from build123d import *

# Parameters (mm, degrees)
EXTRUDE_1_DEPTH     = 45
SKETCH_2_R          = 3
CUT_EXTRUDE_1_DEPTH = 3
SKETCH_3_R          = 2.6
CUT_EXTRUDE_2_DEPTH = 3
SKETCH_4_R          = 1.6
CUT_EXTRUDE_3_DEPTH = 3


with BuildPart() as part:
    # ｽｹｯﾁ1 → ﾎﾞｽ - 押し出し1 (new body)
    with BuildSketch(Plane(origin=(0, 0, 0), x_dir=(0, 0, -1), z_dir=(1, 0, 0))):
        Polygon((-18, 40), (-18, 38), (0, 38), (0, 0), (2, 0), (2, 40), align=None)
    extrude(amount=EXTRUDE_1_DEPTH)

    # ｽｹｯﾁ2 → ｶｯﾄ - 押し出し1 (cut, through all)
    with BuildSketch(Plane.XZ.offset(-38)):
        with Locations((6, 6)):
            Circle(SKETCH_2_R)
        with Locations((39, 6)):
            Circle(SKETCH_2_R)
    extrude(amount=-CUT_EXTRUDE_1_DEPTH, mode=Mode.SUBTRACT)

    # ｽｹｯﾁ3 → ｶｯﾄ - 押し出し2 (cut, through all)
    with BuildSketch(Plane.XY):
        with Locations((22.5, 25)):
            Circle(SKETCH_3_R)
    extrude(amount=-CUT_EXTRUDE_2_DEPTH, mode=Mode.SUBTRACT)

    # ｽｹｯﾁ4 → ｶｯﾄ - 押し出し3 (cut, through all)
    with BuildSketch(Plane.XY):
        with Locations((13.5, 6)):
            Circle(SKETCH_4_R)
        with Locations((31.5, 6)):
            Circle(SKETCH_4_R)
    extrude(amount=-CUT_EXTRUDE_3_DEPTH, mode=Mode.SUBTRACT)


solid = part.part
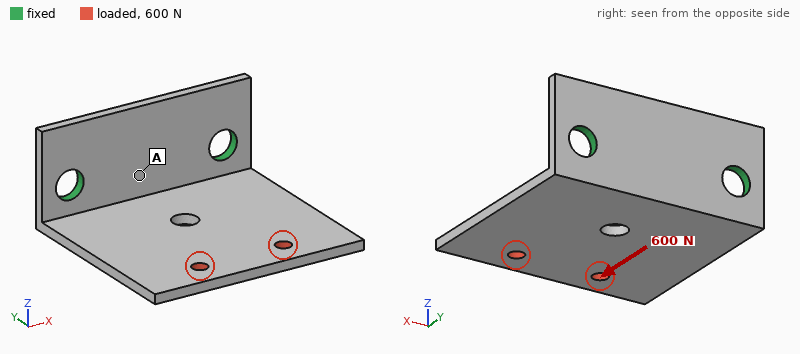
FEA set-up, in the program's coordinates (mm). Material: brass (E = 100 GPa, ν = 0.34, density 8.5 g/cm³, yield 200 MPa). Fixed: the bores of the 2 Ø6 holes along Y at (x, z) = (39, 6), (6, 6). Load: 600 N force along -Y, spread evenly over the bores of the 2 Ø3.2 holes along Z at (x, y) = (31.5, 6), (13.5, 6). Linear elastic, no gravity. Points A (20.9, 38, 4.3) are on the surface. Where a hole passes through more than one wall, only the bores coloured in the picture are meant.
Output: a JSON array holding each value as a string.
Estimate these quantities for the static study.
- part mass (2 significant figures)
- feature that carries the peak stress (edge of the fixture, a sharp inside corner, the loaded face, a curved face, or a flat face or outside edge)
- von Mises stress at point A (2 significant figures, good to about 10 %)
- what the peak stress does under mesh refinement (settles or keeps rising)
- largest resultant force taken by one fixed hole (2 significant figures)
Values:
["43 g", "edge of the fixture", "16 MPa", "keeps rising", "300 N"]
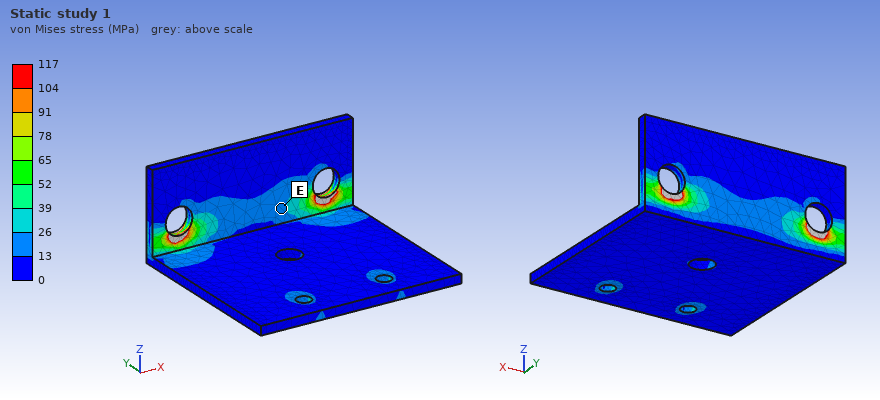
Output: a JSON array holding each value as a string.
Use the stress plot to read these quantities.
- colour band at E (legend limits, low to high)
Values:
["13 to 26 MPa"]
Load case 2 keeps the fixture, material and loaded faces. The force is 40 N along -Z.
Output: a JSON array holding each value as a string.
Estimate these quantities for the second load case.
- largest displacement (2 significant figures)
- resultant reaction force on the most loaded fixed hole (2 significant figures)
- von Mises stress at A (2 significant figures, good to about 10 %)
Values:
["0.28 mm", "20 N", "21 MPa"]
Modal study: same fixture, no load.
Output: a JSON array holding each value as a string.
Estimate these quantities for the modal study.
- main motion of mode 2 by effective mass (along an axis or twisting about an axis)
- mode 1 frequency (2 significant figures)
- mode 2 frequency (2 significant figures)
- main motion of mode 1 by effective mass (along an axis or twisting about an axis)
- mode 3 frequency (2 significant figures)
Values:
["twisting about Y", "620 Hz", "1500 Hz", "along Z", "3700 Hz"]
